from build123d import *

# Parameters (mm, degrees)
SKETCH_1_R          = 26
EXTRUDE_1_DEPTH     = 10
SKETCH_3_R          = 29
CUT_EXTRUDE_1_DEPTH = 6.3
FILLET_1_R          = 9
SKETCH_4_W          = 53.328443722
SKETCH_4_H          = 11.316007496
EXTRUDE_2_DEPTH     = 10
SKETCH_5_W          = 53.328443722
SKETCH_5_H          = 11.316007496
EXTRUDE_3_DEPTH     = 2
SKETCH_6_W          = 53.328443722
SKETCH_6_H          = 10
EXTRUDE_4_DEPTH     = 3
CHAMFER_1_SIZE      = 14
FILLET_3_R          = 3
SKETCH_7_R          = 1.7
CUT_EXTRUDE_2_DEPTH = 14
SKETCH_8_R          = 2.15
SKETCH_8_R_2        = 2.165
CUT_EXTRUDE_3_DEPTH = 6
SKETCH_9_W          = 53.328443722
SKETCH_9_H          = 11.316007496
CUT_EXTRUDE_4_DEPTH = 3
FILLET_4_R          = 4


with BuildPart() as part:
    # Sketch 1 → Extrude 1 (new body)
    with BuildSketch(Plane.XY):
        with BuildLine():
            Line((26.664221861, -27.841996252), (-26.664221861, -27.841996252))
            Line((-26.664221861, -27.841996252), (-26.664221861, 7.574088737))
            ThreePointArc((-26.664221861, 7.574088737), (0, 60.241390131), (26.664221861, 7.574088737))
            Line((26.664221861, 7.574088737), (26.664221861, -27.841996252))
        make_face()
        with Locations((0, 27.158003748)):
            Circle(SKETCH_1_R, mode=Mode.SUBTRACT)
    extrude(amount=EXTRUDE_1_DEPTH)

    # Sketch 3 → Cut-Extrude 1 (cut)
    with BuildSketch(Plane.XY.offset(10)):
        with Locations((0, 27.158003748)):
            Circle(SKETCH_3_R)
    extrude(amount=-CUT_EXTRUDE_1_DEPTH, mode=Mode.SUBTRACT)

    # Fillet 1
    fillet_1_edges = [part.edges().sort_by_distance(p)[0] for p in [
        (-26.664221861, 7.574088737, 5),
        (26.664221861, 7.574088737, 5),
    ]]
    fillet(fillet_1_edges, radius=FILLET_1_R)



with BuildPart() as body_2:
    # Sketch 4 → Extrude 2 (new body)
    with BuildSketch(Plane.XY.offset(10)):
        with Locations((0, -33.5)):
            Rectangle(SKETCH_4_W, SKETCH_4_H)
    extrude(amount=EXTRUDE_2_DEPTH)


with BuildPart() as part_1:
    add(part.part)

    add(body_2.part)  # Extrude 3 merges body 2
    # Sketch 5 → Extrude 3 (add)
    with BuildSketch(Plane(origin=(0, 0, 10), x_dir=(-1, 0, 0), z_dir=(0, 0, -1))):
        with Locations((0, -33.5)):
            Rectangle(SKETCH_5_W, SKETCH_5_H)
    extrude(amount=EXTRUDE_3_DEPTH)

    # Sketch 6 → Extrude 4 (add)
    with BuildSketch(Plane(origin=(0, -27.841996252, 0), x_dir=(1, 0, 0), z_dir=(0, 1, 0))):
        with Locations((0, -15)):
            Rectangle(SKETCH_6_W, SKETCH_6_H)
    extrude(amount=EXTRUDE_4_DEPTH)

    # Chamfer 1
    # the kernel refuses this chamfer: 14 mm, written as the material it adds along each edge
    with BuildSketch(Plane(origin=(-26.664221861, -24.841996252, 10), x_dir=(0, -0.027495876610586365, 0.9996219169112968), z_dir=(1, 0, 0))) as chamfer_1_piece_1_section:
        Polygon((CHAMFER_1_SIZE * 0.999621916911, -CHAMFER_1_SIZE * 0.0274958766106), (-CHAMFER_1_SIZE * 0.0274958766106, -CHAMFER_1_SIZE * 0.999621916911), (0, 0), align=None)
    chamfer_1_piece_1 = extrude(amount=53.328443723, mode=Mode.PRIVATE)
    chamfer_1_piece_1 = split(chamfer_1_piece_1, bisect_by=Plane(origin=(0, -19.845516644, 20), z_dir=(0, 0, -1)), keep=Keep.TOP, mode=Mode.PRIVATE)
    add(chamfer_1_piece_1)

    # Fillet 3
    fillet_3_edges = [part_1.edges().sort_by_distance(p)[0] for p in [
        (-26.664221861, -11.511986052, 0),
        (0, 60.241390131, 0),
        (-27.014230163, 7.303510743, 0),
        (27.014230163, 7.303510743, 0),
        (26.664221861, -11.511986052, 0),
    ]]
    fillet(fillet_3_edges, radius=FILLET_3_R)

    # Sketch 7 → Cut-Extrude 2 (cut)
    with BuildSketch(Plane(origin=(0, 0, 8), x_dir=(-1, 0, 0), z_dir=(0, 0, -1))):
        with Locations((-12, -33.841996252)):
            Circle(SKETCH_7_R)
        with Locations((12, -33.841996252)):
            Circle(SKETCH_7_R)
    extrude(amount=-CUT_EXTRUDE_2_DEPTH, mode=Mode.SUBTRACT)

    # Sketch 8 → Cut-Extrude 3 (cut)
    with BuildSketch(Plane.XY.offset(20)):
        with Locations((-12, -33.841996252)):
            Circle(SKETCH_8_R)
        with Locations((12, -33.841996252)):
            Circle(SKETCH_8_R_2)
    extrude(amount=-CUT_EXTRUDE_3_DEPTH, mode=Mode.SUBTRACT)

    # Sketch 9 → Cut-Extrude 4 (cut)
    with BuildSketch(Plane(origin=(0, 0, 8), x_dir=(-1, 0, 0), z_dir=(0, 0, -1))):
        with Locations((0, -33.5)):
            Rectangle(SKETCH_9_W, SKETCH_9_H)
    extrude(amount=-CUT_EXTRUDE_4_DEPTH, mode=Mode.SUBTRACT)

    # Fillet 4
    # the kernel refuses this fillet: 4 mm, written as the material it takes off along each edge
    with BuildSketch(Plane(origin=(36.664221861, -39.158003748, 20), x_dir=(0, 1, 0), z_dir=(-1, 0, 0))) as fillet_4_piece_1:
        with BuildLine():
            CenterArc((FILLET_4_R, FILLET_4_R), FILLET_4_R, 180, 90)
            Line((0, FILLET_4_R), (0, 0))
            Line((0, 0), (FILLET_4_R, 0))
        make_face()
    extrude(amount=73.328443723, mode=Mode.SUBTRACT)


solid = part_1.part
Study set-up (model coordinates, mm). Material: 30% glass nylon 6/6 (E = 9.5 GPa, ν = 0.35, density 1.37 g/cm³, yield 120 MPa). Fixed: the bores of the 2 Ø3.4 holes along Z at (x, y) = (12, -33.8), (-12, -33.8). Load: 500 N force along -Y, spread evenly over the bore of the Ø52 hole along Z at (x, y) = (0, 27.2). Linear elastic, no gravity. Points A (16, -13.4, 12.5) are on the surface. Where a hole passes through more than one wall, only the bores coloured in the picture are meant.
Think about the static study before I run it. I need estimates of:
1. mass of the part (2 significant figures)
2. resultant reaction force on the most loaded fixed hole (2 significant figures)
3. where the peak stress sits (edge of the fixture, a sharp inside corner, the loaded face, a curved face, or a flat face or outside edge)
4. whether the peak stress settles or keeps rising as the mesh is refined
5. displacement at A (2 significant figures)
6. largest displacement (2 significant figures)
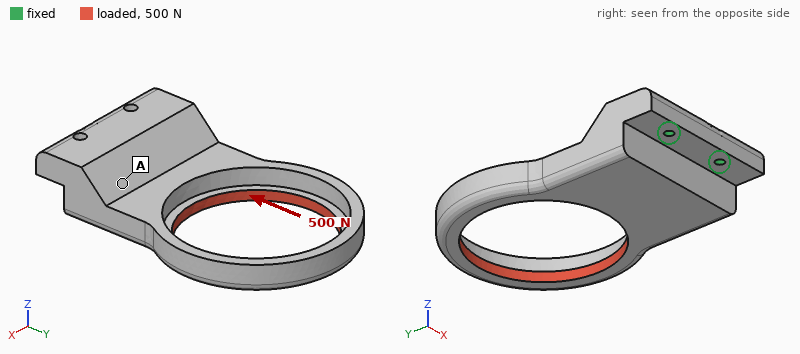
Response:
48 g
250 N
edge of the fixture
keeps rising
0.21 mm
1.3 mm
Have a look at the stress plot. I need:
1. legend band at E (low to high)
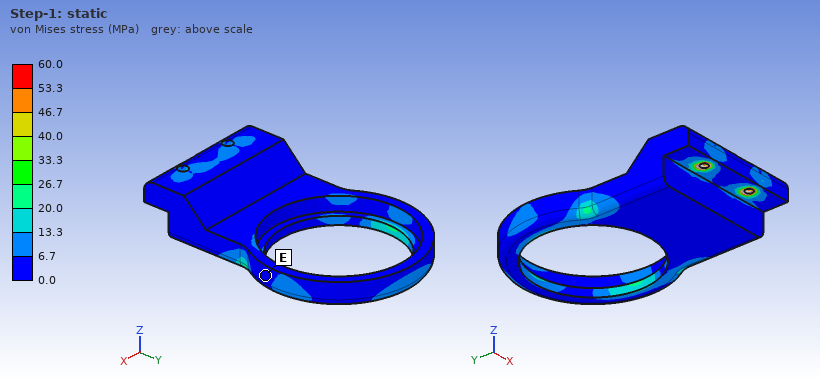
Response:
0.0 to 6.7 MPa
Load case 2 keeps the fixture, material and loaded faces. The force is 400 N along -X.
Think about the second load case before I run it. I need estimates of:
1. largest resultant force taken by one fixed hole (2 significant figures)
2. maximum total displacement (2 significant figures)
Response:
990 N
1.1 mm
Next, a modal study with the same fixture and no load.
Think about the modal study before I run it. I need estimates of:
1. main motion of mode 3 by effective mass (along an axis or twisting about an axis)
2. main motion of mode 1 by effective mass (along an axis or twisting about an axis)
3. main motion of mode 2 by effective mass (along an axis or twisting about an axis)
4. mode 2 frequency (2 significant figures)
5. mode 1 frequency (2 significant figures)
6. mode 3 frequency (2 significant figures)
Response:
along Z
along Z
along X
910 Hz
390 Hz
1400 Hz
